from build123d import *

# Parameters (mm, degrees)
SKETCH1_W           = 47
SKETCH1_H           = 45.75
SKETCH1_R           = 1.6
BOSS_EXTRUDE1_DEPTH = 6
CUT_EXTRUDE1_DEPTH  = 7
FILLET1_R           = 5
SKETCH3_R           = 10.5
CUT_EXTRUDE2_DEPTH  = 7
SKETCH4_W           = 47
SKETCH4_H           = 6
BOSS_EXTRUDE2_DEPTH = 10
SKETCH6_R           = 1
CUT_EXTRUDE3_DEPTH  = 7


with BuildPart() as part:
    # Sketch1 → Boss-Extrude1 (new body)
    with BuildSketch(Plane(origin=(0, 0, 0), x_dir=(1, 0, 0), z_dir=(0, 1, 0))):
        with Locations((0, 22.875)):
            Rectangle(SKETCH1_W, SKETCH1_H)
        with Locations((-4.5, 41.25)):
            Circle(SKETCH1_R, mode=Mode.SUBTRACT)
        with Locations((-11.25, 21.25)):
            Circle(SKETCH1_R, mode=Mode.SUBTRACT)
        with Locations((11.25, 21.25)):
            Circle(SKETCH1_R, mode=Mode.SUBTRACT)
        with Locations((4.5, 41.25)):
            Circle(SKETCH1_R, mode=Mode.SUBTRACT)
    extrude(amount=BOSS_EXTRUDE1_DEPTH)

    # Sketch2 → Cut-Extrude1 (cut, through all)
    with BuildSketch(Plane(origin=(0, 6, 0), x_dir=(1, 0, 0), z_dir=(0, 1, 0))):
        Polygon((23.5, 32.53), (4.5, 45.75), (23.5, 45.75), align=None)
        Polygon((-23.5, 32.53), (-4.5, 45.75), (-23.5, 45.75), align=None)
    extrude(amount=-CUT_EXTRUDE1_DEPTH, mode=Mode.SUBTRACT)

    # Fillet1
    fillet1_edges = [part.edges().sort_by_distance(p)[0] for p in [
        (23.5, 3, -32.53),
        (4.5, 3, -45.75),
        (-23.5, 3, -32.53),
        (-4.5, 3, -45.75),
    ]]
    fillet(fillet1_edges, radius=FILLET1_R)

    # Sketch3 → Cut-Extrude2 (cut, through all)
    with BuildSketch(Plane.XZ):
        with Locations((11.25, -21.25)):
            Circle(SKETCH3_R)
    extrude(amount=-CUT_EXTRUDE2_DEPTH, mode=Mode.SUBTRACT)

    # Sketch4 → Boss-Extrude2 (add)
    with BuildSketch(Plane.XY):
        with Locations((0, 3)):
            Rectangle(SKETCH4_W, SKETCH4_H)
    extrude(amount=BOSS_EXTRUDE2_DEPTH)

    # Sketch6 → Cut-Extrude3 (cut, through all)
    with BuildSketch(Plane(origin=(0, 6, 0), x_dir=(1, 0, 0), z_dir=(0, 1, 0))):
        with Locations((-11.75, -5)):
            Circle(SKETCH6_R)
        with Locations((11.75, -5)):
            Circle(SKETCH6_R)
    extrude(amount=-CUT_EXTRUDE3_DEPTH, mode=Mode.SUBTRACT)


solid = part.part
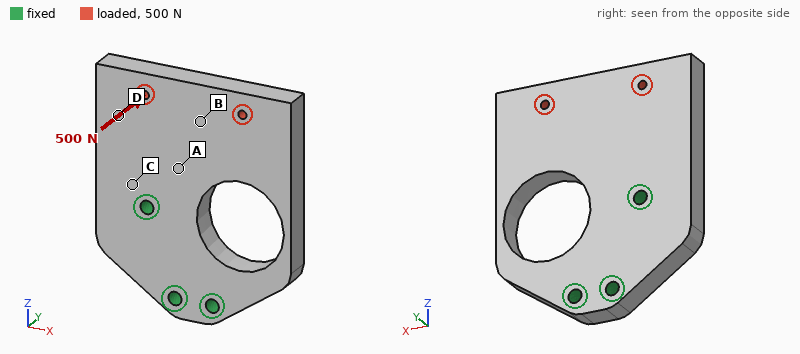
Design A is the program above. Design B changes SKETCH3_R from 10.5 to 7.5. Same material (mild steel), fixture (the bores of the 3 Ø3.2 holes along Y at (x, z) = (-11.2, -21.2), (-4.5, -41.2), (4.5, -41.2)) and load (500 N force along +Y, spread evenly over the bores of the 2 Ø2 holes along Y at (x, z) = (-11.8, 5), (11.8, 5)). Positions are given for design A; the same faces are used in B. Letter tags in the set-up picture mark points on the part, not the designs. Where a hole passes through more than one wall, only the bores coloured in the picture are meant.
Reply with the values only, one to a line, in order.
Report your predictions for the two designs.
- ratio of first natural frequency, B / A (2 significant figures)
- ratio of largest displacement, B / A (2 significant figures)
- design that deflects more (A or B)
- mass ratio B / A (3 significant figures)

1.1
0.84
A
1.09
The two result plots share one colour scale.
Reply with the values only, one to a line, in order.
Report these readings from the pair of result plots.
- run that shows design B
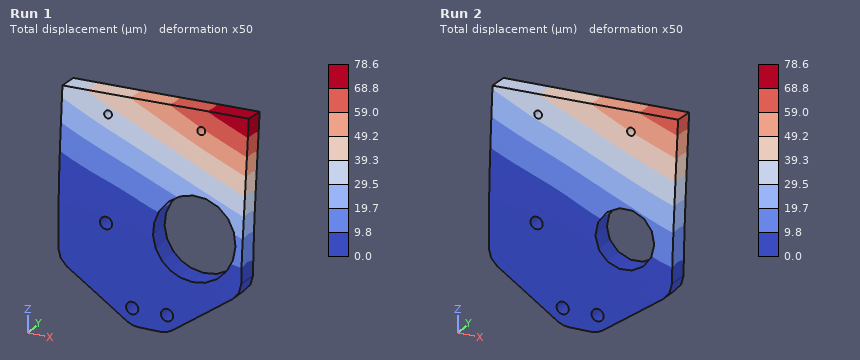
Run 2
